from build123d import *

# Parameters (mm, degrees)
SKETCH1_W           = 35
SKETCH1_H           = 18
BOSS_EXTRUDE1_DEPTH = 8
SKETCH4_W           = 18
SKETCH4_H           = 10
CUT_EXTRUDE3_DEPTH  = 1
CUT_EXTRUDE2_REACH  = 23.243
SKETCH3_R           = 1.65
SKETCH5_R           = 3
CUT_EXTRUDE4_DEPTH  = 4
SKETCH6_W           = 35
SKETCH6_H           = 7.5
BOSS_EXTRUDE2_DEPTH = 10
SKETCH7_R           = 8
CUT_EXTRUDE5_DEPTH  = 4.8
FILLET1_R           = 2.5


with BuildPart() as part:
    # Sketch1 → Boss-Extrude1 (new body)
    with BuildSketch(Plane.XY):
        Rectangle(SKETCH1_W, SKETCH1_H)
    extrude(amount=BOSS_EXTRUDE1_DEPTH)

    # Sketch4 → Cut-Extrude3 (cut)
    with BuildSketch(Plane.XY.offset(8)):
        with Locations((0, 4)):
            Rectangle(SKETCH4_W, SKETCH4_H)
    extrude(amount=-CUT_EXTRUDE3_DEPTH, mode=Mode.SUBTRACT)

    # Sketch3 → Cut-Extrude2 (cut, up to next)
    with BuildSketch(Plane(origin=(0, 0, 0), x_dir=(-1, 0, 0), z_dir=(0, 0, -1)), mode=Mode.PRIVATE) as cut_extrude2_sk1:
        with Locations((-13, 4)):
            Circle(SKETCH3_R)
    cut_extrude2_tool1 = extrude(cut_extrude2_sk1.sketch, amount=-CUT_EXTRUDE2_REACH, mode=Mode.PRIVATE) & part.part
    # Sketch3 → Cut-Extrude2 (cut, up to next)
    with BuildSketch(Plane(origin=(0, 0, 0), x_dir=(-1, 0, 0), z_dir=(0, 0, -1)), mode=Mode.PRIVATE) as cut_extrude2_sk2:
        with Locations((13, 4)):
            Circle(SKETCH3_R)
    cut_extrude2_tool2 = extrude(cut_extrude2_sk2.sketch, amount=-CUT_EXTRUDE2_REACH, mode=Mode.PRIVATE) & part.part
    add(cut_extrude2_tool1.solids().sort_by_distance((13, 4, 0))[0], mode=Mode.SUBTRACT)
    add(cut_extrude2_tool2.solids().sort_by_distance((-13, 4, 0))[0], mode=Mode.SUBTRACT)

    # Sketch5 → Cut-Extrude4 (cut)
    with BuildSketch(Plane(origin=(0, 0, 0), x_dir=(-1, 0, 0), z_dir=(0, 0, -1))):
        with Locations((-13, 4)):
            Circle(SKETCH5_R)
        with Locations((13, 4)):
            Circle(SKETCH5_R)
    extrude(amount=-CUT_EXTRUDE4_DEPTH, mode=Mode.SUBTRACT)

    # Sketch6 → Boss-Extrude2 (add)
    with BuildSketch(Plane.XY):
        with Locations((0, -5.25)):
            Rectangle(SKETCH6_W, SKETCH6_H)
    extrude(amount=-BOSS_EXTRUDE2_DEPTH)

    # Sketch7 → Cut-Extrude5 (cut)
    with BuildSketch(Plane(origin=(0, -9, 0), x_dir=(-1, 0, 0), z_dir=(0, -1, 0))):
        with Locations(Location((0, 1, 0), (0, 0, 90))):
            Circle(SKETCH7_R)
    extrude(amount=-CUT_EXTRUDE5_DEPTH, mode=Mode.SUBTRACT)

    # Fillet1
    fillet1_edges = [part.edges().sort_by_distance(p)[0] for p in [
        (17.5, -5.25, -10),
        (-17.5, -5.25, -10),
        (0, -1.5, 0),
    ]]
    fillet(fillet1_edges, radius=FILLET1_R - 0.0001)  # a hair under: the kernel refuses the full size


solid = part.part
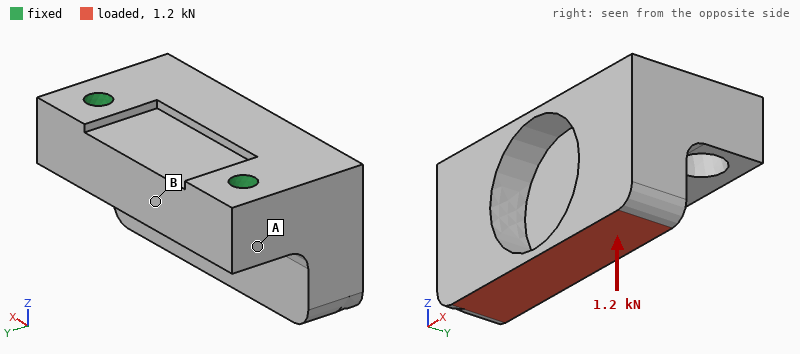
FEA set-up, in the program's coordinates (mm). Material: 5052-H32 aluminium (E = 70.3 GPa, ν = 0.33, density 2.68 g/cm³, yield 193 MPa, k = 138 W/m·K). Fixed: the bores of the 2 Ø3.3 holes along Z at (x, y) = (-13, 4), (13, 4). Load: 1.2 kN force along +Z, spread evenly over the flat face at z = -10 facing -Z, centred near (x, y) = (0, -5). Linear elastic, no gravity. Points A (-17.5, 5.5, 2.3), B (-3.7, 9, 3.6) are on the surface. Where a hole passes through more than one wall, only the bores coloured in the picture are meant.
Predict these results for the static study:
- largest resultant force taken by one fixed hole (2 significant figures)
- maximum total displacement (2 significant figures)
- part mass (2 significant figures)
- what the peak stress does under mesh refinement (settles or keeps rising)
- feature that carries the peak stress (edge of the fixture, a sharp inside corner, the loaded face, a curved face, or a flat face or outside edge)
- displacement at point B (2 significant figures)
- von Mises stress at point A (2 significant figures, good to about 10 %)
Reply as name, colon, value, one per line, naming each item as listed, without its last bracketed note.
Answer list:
largest resultant force taken by one fixed hole: 600 N
maximum total displacement: 58 µm
part mass: 17 g
what the peak stress does under mesh refinement: keeps rising
feature that carries the peak stress: edge of the fixture
displacement at point B: 9.3 µm
von Mises stress at point A: 31 MPa
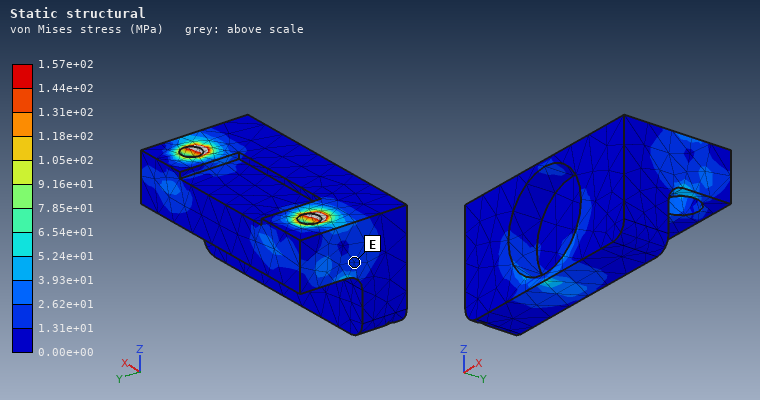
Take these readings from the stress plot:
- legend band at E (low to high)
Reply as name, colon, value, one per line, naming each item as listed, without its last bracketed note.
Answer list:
legend band at E: 1.31e+01 to 2.62e+01 MPa
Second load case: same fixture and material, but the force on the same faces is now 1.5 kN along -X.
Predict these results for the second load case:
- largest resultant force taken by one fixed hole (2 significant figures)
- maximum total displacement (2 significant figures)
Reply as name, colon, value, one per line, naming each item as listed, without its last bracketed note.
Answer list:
largest resultant force taken by one fixed hole: 1.2 kN
maximum total displacement: 18 µm
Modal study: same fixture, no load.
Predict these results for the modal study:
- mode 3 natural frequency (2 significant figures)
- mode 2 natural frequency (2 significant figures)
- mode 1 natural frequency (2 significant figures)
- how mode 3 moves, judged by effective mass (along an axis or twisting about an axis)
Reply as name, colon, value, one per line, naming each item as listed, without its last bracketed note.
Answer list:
mode 3 natural frequency: 24 kHz
mode 2 natural frequency: 15 kHz
mode 1 natural frequency: 8300 Hz
how mode 3 moves, judged by effective mass: along X
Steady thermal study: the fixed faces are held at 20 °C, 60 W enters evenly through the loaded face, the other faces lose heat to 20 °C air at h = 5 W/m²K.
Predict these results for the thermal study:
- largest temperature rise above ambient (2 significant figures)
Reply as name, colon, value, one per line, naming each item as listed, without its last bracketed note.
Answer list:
largest temperature rise above ambient: 65 K
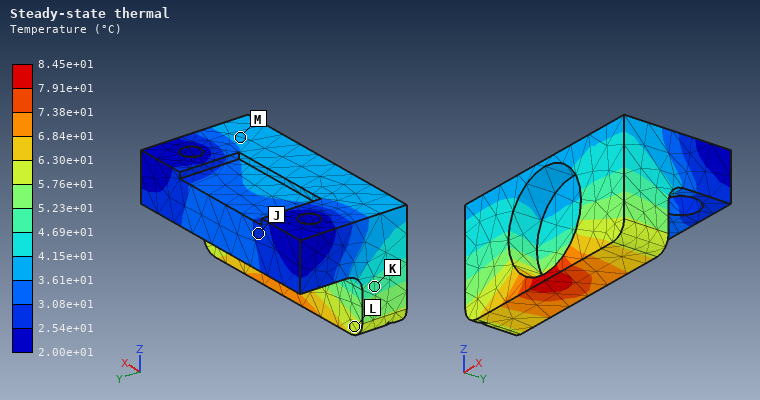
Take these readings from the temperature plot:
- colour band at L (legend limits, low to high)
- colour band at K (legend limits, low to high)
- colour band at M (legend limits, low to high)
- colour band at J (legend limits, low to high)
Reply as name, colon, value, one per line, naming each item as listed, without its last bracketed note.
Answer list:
colour band at L: 5.76e+01 to 6.30e+01 °C
colour band at K: 4.69e+01 to 5.23e+01 °C
colour band at M: 3.61e+01 to 4.15e+01 °C
colour band at J: 2.54e+01 to 3.08e+01 °C
